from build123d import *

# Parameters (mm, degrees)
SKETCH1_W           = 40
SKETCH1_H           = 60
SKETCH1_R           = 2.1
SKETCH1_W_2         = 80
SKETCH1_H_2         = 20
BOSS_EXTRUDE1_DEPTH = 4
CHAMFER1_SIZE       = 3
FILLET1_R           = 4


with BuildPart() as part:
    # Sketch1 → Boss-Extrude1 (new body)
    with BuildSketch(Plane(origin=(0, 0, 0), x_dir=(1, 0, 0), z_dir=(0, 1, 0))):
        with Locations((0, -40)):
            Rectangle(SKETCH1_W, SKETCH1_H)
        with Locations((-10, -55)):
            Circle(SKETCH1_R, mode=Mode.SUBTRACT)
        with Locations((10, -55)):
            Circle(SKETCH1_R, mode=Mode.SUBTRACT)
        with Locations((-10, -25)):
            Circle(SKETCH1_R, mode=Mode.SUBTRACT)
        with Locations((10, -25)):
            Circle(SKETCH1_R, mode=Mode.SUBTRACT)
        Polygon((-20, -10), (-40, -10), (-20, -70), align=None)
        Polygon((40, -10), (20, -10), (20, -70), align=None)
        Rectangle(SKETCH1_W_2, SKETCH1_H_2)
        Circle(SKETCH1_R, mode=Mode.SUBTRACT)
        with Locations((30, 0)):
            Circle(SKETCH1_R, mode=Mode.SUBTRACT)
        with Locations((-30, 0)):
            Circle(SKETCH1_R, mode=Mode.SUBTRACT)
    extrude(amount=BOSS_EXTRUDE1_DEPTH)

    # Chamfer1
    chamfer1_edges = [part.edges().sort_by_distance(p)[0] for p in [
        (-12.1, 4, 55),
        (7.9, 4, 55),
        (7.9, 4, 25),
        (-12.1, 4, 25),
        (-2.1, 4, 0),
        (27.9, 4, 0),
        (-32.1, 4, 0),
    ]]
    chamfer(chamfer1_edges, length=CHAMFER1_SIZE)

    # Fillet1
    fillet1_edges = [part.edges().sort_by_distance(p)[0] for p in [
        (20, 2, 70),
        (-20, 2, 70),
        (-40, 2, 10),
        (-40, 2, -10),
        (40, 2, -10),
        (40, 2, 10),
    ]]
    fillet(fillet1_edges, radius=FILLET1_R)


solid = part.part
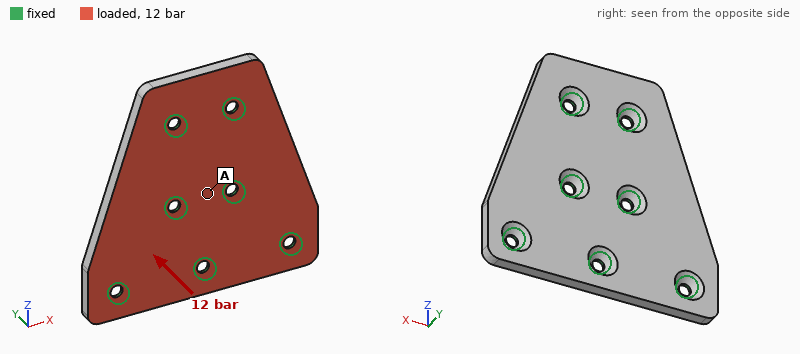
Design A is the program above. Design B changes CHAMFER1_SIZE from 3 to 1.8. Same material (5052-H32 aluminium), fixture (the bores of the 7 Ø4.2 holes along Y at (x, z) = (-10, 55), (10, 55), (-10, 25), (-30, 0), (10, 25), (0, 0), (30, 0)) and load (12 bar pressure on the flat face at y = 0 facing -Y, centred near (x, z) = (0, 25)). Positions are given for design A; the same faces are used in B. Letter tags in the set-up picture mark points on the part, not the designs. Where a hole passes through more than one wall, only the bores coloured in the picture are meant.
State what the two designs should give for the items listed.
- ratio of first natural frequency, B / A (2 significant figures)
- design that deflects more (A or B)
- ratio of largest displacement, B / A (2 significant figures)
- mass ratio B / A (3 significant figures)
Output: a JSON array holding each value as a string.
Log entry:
["1.1", "A", "0.83", "1.02"]
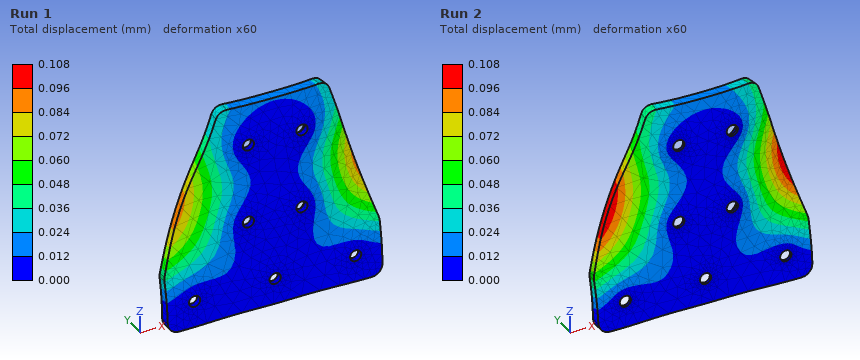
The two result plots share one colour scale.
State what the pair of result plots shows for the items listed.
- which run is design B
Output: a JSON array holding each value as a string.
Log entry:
["Run 1"]
